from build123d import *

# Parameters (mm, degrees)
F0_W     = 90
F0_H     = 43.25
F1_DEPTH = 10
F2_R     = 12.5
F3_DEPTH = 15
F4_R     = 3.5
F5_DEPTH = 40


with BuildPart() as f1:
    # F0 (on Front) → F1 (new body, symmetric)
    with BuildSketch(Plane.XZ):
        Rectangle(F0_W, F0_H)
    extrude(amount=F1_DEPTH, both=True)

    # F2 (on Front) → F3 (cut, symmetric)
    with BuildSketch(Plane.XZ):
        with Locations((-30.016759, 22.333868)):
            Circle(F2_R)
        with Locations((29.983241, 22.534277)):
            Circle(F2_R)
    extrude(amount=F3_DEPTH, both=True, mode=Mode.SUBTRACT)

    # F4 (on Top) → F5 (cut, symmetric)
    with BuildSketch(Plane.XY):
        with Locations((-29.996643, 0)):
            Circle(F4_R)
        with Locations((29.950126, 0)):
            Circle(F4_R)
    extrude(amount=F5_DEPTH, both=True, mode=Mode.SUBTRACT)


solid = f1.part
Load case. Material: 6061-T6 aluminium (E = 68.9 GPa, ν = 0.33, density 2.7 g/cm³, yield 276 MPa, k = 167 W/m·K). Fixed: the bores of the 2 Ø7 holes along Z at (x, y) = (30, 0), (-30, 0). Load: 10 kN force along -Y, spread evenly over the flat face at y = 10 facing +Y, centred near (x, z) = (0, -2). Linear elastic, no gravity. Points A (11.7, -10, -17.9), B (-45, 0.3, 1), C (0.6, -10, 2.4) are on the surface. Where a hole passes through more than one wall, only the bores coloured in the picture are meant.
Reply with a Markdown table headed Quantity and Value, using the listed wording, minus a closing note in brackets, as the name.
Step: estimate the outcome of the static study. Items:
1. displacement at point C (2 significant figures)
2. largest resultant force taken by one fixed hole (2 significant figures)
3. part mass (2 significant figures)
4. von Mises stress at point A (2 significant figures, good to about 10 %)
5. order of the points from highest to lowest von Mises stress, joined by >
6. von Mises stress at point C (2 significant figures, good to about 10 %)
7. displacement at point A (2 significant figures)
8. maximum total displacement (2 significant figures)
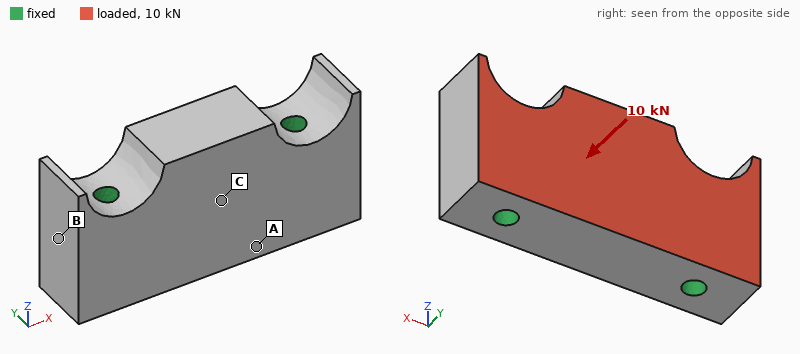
| Quantity | Value |
|---|---|
| displacement at point C | 6.7 µm |
| largest resultant force taken by one fixed hole | 5.0 kN |
| part mass | 180 g |
| von Mises stress at point A | 5.6 MPa |
| order of the points from highest to lowest von Mises stress, joined by > | C > A > B |
| von Mises stress at point C | 9.3 MPa |
| displacement at point A | 4.2 µm |
| maximum total displacement | 11 µm |
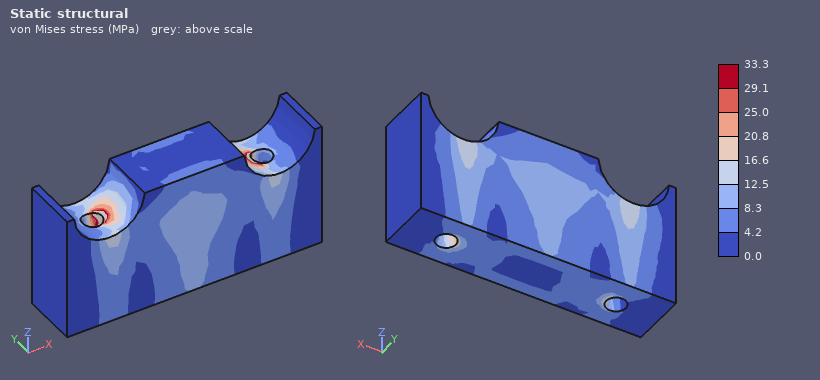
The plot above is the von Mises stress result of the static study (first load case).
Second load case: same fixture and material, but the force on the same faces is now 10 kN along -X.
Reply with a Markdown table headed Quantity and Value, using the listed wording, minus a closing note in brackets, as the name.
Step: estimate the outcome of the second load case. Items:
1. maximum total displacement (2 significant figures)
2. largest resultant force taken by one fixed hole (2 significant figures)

| Quantity | Value |
|---|---|
| maximum total displacement | 8.2 µm |
| largest resultant force taken by one fixed hole | 5.2 kN |
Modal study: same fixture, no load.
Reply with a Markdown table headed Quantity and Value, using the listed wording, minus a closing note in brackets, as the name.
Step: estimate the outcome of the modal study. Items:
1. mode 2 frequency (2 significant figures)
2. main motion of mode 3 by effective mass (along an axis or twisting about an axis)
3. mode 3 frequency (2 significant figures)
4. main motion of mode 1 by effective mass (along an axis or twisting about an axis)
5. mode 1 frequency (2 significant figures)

| Quantity | Value |
|---|---|
| mode 2 frequency | 19 kHz |
| main motion of mode 3 by effective mass | along Z |
| mode 3 frequency | 21 kHz |
| main motion of mode 1 by effective mass | along Y |
| mode 1 frequency | 13 kHz |
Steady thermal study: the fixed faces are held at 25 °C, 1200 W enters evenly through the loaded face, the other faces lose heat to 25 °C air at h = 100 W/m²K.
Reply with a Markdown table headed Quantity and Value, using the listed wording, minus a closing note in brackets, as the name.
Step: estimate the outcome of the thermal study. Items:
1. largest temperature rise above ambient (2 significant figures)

| Quantity | Value |
|---|---|
| largest temperature rise above ambient | 73 K |
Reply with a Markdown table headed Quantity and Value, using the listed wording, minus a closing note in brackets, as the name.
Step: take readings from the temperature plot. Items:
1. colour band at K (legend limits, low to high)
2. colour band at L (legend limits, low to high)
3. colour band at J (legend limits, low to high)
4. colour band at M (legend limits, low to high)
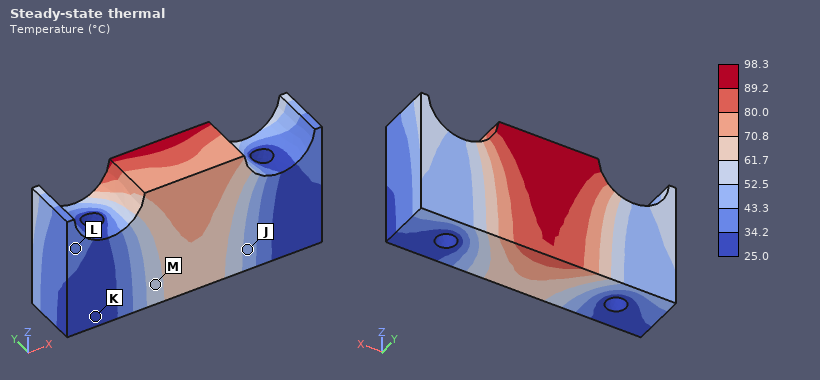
| Quantity | Value |
|---|---|
| colour band at K | 25.0 to 34.2 °C |
| colour band at L | 34.2 to 43.3 °C |
| colour band at J | 43.3 to 52.5 °C |
| colour band at M | 52.5 to 61.7 °C |
